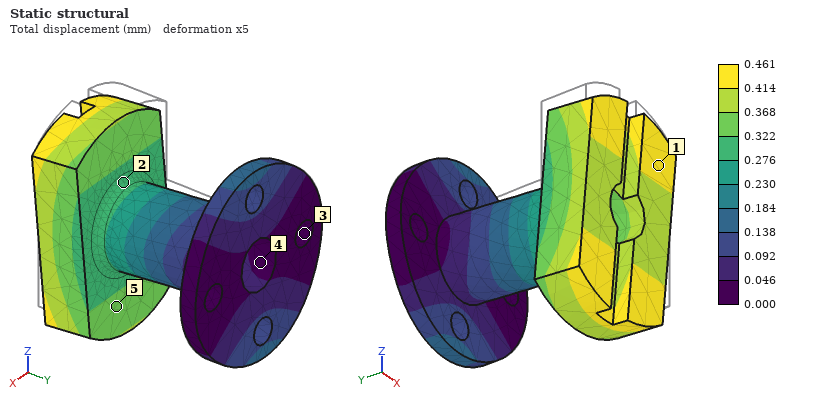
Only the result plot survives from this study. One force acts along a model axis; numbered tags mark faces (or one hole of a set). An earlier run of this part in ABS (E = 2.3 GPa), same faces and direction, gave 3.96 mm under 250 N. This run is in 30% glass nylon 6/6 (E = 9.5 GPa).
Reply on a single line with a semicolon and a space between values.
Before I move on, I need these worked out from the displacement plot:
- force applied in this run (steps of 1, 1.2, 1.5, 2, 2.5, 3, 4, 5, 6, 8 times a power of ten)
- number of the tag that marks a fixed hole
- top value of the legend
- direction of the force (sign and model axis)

120 N; 3; 0.461 mm; -Z
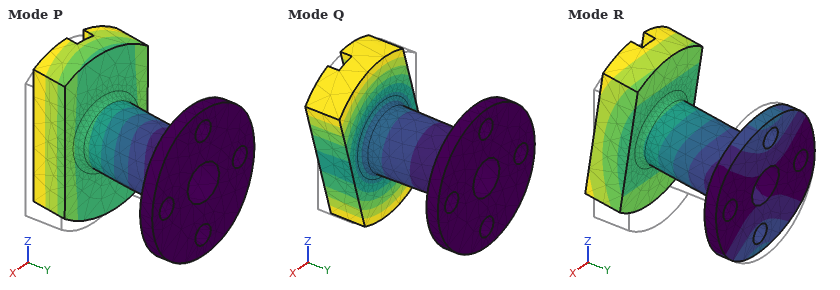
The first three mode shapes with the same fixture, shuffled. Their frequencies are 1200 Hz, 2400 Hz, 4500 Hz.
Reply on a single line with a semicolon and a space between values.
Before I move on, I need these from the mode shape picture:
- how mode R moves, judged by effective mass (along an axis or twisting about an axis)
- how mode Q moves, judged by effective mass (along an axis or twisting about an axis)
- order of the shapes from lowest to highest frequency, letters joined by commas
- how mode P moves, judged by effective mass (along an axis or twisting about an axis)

along Z; twisting about Y; R, P, Q; along X
